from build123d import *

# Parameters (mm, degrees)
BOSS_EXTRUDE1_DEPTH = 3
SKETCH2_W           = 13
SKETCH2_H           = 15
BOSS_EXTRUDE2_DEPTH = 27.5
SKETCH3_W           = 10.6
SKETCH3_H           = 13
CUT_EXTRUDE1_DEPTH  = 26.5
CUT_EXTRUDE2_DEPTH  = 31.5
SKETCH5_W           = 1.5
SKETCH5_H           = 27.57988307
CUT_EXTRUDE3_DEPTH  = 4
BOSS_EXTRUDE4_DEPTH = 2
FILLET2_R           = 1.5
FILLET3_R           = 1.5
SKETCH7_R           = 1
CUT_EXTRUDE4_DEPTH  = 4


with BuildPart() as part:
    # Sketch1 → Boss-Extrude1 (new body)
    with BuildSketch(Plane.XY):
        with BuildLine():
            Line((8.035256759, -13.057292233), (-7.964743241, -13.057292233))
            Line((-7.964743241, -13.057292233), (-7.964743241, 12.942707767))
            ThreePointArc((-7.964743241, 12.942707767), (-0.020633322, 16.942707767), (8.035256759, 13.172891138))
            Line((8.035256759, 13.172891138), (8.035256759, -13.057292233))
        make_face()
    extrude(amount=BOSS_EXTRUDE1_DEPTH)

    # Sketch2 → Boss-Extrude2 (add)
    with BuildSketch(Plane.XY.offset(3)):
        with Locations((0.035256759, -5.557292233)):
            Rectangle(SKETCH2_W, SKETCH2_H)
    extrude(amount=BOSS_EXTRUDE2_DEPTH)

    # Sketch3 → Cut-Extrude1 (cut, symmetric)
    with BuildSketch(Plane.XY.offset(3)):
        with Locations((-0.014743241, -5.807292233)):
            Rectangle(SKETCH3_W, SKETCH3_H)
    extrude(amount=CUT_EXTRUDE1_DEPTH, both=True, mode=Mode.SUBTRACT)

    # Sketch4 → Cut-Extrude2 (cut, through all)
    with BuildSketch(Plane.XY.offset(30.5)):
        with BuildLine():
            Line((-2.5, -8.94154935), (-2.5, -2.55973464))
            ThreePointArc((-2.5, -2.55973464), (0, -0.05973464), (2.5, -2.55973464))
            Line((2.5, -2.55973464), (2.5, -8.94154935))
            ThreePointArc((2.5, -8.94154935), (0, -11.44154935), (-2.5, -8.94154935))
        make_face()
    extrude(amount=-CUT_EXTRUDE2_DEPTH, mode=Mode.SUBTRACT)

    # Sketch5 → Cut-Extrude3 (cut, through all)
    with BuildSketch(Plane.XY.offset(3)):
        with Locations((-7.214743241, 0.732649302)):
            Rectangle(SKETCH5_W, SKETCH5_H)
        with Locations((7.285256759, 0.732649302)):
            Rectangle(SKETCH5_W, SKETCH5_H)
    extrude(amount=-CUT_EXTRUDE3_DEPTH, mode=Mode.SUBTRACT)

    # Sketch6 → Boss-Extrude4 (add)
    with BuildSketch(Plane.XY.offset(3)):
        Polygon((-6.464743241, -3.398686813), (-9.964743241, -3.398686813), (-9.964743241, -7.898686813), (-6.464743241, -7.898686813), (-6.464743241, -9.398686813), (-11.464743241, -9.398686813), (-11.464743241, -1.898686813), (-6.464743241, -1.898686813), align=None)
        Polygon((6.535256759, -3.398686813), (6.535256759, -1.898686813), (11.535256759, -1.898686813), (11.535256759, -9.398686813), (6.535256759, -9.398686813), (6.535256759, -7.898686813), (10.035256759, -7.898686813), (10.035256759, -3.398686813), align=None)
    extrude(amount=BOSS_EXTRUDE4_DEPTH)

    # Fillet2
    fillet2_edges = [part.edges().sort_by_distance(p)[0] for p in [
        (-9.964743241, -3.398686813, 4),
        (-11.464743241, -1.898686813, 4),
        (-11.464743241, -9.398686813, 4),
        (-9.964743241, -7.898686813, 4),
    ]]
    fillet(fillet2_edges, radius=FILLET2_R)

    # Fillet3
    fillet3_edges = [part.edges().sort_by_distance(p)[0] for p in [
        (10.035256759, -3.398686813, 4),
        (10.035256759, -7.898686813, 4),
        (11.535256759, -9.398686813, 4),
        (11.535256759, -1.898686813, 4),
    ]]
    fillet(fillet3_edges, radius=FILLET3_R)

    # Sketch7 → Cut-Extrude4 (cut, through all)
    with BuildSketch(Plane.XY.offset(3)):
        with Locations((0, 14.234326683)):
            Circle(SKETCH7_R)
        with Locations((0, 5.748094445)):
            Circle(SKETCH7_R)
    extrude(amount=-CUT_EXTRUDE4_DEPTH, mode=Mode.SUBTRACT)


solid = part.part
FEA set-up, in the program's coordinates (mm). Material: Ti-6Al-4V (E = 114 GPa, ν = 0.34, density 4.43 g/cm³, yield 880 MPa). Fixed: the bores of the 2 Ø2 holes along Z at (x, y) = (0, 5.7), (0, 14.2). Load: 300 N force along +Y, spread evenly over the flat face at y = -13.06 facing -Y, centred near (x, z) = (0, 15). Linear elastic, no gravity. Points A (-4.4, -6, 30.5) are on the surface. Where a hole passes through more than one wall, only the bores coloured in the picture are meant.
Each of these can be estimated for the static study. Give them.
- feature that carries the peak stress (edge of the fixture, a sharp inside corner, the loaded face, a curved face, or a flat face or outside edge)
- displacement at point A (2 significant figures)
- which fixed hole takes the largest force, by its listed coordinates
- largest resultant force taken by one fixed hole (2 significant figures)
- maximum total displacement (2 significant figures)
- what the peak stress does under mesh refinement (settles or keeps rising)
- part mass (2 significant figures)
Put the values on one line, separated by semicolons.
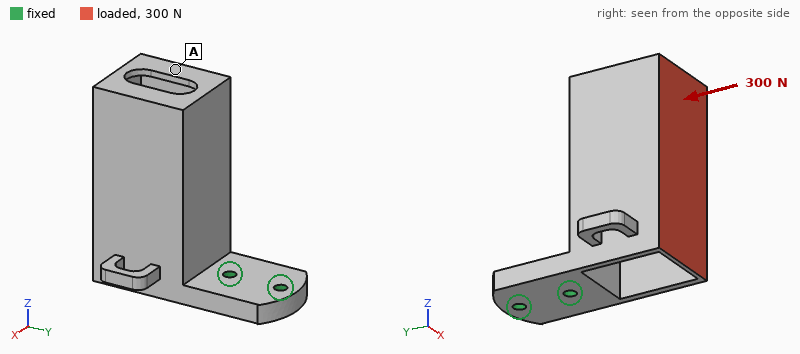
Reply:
edge of the fixture; 0.41 mm; (0, 5.7); 310 N; 0.45 mm; keeps rising; 11 g
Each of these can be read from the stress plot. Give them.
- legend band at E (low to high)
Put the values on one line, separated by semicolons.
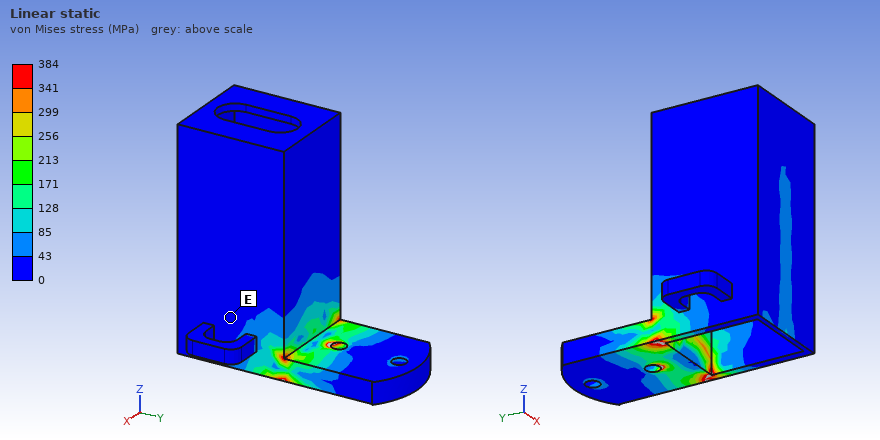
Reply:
0 to 43 MPa
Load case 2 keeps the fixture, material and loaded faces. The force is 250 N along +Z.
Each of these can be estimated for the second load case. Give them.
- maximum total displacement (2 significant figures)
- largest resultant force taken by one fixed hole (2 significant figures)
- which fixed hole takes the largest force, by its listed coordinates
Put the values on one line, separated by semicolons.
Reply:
0.43 mm; 480 N; (0, 5.7)
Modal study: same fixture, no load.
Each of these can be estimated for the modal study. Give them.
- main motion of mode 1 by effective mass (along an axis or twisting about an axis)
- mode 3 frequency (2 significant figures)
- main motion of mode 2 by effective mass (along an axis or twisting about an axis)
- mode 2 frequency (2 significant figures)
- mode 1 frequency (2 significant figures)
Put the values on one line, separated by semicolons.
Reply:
along Y; 4100 Hz; along X; 2600 Hz; 1600 Hz
